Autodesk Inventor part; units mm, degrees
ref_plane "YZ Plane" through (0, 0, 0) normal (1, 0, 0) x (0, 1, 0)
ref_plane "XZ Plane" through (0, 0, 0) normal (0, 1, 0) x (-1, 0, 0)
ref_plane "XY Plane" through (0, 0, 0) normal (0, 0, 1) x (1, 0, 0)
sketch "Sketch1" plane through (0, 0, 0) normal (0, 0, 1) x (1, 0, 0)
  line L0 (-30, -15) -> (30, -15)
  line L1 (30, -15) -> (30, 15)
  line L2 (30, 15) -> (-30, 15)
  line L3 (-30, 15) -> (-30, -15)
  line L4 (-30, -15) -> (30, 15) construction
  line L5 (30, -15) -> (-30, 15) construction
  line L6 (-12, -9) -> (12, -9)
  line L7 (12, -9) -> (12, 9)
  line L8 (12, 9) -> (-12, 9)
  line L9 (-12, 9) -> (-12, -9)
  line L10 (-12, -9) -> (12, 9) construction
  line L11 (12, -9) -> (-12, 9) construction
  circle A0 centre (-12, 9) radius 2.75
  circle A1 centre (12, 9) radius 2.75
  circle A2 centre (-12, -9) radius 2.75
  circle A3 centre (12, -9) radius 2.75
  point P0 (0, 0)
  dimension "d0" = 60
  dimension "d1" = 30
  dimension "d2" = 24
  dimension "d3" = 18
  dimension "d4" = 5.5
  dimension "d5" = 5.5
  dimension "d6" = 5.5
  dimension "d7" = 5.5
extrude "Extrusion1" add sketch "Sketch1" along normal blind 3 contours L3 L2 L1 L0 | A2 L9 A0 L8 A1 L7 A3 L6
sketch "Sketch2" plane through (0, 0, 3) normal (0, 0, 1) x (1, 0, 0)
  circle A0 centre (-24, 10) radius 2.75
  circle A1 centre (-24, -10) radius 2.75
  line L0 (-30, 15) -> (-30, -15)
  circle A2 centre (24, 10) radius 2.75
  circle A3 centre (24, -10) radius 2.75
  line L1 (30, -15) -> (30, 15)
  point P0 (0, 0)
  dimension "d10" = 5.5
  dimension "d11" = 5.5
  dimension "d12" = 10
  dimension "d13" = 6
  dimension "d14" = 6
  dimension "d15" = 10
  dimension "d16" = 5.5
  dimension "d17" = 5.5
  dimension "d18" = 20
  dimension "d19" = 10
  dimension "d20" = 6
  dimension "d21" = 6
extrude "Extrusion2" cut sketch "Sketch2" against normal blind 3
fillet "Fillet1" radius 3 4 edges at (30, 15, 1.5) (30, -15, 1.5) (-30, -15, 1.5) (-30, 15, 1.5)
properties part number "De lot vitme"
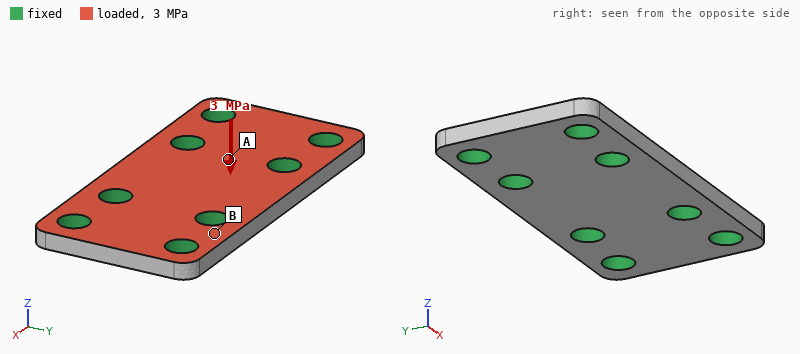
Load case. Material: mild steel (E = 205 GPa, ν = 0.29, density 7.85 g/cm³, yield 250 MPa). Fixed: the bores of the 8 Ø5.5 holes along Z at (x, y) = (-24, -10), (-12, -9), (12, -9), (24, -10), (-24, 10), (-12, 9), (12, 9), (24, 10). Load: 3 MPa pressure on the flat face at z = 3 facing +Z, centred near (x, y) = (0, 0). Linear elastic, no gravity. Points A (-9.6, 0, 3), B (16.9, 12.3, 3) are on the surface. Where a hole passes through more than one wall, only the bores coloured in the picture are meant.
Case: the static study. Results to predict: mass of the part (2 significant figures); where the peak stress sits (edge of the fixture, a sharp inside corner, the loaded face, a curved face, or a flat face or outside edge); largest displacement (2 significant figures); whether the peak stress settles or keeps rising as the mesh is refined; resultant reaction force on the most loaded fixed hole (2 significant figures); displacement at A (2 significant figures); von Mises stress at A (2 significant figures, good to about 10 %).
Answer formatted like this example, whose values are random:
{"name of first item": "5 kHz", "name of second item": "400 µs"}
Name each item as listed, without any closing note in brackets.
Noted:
{"mass of the part": "38 g", "where the peak stress sits": "edge of the fixture", "largest displacement": "4.8 µm", "whether the peak stress settles or keeps rising as the mesh is refined": "keeps rising", "resultant reaction force on the most loaded fixed hole": "750 N", "displacement at A": "2.0 µm", "von Mises stress at A": "28 MPa"}
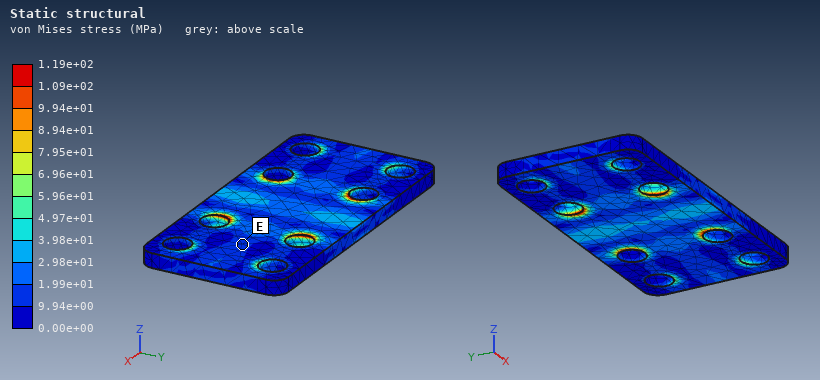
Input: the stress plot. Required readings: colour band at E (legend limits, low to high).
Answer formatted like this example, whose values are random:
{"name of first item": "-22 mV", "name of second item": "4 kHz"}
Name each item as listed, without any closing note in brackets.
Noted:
{"colour band at E": "9.94e+00 to 1.99e+01 MPa"}
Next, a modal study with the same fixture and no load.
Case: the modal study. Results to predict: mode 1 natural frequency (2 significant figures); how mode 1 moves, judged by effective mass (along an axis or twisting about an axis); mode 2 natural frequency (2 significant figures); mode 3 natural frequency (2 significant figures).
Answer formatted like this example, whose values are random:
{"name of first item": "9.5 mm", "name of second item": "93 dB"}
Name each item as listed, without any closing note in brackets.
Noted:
{"mode 1 natural frequency": "31 kHz", "how mode 1 moves, judged by effective mass": "along Z", "mode 2 natural frequency": "35 kHz", "mode 3 natural frequency": "40 kHz"}
